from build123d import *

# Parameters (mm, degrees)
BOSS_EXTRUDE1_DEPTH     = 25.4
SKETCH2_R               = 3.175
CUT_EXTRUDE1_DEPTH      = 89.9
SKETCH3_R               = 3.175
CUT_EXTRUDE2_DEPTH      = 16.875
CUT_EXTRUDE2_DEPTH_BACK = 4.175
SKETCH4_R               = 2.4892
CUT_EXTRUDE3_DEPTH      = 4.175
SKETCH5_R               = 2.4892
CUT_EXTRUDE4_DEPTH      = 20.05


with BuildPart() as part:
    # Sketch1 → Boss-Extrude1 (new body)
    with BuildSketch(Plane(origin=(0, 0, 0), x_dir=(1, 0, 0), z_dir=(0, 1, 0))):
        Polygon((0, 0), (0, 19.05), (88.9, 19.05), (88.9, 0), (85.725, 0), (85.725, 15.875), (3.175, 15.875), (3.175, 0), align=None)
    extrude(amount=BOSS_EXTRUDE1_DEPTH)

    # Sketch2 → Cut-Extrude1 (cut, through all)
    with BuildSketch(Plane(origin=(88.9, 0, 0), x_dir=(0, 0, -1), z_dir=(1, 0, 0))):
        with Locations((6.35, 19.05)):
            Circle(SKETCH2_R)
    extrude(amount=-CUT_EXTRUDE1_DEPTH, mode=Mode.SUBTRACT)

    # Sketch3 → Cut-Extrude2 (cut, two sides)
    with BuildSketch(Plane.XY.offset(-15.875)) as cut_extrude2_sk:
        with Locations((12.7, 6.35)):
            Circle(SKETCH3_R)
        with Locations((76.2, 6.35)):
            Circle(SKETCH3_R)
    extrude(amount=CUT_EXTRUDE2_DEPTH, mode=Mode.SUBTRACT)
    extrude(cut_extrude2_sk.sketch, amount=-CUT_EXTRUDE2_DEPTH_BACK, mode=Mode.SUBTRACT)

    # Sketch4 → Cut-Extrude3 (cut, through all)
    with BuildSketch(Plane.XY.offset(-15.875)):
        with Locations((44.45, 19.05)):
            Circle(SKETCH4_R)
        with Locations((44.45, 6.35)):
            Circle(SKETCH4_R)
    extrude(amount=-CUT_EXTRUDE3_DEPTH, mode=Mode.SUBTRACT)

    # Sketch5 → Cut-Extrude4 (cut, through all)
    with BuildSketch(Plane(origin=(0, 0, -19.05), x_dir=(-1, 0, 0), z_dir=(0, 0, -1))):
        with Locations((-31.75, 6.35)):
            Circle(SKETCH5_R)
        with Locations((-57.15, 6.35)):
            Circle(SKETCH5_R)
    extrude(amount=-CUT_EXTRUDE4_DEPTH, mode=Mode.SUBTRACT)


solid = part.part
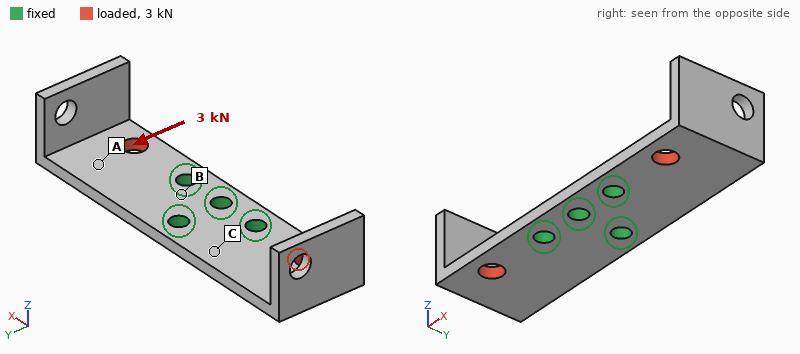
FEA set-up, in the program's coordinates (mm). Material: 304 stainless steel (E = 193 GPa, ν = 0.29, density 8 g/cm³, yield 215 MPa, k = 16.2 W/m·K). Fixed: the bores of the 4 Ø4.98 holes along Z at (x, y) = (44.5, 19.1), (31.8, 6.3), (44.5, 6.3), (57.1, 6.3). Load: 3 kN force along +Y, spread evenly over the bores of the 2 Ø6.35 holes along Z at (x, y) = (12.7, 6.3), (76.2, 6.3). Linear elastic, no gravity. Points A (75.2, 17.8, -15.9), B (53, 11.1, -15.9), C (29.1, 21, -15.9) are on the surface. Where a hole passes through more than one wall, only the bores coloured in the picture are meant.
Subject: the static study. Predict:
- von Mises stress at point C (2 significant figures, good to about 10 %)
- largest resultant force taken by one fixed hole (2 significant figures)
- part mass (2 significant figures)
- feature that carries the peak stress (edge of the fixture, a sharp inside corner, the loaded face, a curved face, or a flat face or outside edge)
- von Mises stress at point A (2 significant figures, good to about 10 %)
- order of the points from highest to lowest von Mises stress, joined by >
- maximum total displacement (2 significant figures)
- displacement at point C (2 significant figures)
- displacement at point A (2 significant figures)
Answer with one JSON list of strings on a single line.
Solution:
["44 MPa", "2.2 kN", "73 g", "edge of the fixture", "28 MPa", "C > A > B", "23 µm", "4.1 µm", "13 µm"]
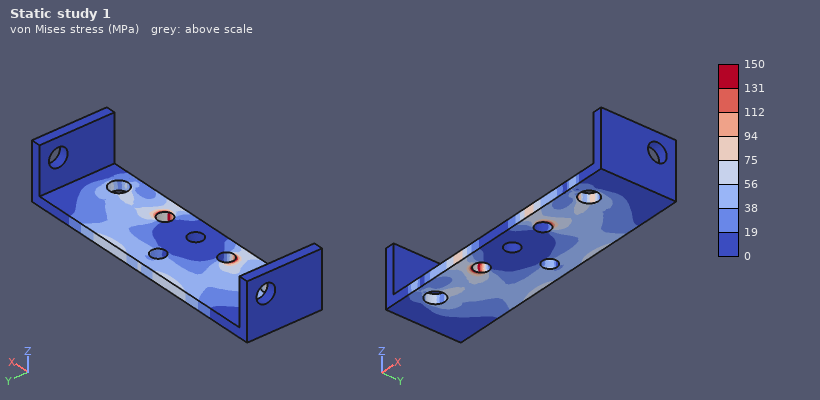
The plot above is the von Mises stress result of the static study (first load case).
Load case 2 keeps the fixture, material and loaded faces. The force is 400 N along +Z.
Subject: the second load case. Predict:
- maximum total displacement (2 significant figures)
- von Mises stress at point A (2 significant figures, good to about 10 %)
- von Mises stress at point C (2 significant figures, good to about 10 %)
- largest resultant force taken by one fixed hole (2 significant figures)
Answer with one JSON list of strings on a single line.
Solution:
["88 µm", "18 MPa", "36 MPa", "280 N"]
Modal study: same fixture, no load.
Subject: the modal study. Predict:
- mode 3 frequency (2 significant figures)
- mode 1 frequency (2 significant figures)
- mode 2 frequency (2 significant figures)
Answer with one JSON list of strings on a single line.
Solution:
["2900 Hz", "1400 Hz", "1400 Hz"]
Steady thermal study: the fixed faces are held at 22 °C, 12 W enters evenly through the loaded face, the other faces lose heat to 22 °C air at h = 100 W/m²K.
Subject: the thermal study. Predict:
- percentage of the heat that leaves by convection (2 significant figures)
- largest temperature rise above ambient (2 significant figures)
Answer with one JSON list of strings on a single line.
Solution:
["73 %", "51 K"]
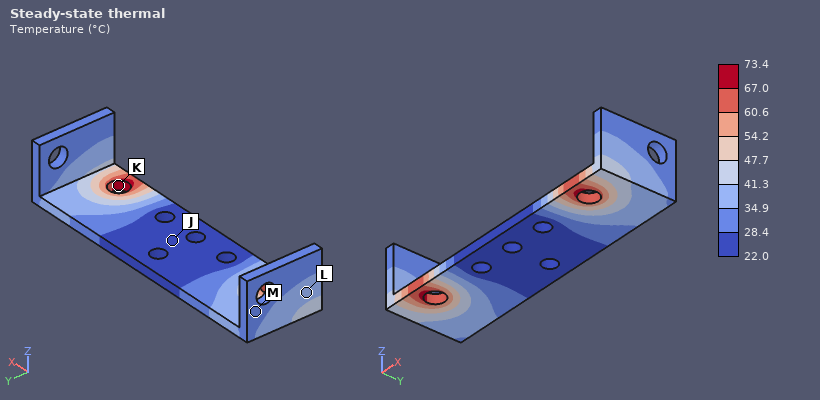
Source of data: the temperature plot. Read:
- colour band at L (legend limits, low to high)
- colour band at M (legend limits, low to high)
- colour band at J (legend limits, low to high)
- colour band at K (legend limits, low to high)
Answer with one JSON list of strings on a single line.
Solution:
["34.9 to 41.3 °C", "28.4 to 34.9 °C", "22.0 to 28.4 °C", "67.0 to 73.4 °C"]
